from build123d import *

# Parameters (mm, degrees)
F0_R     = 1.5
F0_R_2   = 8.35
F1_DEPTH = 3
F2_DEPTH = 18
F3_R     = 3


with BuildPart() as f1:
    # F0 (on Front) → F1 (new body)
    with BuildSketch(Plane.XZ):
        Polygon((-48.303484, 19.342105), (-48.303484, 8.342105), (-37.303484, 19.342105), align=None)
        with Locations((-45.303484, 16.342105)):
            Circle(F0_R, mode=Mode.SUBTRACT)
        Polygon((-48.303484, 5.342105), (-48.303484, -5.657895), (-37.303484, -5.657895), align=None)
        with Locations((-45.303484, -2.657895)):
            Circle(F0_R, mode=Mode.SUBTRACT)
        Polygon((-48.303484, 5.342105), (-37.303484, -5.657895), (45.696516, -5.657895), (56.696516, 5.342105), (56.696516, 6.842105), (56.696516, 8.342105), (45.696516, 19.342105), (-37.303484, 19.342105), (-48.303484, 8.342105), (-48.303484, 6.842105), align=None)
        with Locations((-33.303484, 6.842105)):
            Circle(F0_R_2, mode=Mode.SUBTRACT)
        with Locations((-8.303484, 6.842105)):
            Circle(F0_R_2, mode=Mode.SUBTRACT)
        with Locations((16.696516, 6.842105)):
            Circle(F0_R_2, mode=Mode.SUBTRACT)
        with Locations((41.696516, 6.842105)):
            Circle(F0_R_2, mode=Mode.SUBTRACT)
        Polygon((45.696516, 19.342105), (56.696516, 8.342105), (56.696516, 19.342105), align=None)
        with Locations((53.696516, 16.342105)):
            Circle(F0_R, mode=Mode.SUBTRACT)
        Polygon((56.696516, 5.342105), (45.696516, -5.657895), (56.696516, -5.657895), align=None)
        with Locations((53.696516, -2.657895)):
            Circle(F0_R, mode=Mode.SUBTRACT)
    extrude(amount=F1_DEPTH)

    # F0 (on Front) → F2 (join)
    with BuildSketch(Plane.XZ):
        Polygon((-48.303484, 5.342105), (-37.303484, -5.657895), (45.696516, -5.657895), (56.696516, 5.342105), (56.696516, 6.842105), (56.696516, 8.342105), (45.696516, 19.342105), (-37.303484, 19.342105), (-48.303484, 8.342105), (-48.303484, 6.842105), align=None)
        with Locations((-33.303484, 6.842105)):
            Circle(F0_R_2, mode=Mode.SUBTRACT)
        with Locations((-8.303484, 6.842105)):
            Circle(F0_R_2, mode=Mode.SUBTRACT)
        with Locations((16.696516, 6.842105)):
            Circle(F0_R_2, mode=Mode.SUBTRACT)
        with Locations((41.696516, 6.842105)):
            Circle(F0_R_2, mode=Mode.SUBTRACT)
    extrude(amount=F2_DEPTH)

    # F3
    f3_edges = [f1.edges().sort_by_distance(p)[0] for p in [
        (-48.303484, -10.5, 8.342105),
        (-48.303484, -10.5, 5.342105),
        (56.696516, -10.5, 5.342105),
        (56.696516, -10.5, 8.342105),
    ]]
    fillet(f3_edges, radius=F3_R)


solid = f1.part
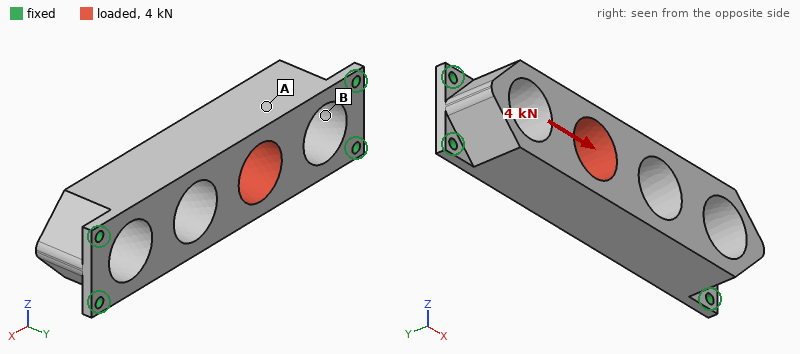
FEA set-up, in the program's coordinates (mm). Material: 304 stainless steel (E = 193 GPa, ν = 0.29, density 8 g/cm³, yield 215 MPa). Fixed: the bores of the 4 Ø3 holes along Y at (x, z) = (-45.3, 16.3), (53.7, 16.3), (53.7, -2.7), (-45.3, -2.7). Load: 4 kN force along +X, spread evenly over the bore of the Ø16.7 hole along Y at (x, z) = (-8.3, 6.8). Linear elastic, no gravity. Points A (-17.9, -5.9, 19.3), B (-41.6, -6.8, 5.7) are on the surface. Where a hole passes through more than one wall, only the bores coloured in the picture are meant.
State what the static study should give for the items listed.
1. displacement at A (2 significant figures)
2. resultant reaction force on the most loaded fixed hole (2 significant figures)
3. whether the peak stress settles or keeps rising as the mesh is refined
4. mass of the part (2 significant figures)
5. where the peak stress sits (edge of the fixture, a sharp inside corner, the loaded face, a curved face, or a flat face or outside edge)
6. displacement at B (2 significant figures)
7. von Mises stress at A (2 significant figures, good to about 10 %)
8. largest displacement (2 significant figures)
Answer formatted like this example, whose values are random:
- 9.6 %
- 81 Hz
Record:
- 5.8 µm
- 1.1 kN
- keeps rising
- 220 g
- edge of the fixture
- 2.5 µm
- 15 MPa
- 6.8 µm
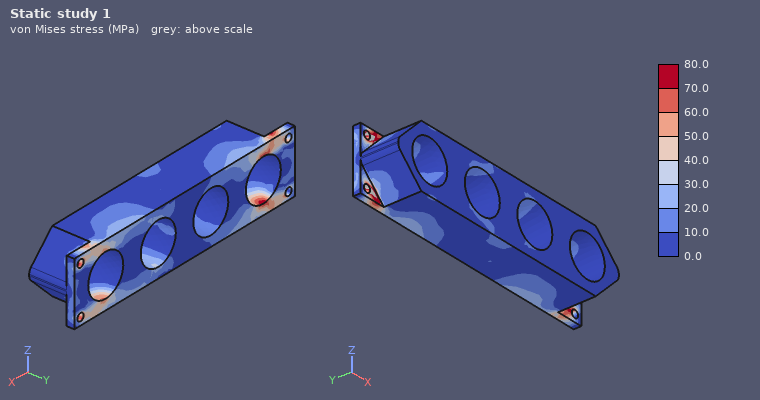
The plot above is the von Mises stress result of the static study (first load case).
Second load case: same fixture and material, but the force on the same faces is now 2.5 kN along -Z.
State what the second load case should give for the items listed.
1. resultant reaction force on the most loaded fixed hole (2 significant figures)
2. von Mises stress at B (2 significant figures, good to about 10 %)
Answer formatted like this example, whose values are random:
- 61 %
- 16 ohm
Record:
- 1.2 kN
- 33 MPa
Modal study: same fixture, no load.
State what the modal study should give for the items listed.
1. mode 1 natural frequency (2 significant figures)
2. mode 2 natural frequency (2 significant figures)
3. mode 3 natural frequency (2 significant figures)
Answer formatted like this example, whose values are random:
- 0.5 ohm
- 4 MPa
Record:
- 4300 Hz
- 4300 Hz
- 6400 Hz
